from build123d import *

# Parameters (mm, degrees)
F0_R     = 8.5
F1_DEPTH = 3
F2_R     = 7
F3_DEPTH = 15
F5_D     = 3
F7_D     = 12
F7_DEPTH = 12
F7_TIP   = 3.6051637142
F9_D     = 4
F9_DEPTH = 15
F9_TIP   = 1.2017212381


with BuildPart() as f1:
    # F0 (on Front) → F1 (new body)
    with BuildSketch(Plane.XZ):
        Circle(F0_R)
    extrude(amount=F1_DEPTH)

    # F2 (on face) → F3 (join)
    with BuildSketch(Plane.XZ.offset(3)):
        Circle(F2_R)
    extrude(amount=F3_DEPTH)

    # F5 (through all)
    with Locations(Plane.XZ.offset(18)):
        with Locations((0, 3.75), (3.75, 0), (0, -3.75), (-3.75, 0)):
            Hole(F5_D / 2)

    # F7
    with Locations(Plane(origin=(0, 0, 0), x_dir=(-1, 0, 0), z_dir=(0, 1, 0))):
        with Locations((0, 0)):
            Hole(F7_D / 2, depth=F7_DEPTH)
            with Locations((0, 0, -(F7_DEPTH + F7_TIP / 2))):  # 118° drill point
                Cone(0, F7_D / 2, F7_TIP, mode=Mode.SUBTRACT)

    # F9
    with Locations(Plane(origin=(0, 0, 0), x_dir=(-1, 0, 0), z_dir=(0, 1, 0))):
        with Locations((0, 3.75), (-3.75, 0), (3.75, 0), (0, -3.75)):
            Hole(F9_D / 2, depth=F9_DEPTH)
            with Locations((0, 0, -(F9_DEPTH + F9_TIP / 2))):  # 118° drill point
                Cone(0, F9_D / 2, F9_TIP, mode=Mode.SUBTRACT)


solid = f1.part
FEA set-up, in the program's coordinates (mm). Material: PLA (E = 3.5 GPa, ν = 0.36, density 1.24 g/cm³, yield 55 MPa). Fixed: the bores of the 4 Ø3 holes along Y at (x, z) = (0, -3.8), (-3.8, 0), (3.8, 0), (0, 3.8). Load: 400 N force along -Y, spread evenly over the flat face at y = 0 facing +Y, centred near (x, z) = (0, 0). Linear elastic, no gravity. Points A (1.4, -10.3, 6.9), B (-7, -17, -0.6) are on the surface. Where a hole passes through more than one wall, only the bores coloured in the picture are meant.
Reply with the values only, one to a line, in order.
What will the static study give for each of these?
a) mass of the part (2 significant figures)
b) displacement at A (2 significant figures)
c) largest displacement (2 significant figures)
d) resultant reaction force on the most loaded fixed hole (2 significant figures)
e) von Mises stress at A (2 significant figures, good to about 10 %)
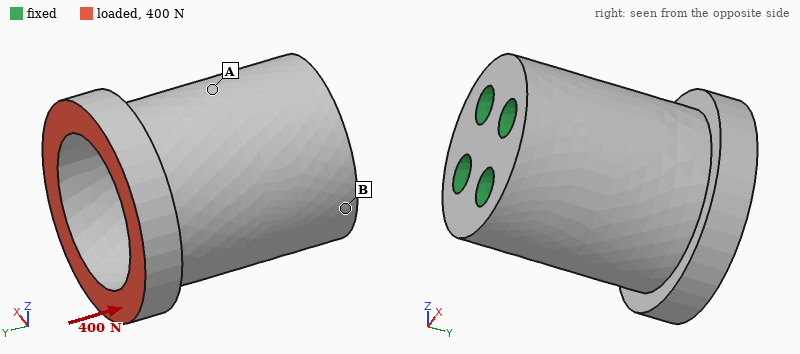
1.6 g
22 µm
57 µm
100 N
9.8 MPa
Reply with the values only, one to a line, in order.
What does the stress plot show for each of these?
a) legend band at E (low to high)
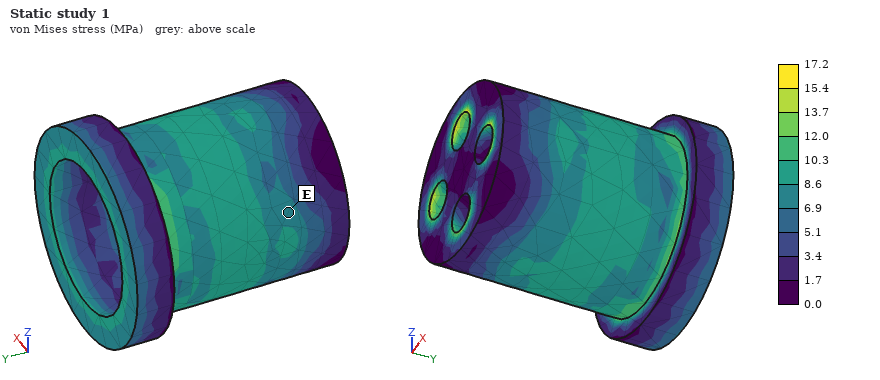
6.9 to 8.6 MPa
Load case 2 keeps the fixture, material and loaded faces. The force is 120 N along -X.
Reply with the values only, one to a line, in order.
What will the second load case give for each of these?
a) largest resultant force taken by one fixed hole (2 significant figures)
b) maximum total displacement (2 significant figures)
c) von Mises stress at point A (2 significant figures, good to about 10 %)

150 N
0.17 mm
9.5 MPa
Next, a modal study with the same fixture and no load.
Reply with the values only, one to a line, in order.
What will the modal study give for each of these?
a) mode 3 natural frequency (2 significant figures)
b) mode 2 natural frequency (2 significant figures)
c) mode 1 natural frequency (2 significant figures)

9300 Hz
6400 Hz
6400 Hz
